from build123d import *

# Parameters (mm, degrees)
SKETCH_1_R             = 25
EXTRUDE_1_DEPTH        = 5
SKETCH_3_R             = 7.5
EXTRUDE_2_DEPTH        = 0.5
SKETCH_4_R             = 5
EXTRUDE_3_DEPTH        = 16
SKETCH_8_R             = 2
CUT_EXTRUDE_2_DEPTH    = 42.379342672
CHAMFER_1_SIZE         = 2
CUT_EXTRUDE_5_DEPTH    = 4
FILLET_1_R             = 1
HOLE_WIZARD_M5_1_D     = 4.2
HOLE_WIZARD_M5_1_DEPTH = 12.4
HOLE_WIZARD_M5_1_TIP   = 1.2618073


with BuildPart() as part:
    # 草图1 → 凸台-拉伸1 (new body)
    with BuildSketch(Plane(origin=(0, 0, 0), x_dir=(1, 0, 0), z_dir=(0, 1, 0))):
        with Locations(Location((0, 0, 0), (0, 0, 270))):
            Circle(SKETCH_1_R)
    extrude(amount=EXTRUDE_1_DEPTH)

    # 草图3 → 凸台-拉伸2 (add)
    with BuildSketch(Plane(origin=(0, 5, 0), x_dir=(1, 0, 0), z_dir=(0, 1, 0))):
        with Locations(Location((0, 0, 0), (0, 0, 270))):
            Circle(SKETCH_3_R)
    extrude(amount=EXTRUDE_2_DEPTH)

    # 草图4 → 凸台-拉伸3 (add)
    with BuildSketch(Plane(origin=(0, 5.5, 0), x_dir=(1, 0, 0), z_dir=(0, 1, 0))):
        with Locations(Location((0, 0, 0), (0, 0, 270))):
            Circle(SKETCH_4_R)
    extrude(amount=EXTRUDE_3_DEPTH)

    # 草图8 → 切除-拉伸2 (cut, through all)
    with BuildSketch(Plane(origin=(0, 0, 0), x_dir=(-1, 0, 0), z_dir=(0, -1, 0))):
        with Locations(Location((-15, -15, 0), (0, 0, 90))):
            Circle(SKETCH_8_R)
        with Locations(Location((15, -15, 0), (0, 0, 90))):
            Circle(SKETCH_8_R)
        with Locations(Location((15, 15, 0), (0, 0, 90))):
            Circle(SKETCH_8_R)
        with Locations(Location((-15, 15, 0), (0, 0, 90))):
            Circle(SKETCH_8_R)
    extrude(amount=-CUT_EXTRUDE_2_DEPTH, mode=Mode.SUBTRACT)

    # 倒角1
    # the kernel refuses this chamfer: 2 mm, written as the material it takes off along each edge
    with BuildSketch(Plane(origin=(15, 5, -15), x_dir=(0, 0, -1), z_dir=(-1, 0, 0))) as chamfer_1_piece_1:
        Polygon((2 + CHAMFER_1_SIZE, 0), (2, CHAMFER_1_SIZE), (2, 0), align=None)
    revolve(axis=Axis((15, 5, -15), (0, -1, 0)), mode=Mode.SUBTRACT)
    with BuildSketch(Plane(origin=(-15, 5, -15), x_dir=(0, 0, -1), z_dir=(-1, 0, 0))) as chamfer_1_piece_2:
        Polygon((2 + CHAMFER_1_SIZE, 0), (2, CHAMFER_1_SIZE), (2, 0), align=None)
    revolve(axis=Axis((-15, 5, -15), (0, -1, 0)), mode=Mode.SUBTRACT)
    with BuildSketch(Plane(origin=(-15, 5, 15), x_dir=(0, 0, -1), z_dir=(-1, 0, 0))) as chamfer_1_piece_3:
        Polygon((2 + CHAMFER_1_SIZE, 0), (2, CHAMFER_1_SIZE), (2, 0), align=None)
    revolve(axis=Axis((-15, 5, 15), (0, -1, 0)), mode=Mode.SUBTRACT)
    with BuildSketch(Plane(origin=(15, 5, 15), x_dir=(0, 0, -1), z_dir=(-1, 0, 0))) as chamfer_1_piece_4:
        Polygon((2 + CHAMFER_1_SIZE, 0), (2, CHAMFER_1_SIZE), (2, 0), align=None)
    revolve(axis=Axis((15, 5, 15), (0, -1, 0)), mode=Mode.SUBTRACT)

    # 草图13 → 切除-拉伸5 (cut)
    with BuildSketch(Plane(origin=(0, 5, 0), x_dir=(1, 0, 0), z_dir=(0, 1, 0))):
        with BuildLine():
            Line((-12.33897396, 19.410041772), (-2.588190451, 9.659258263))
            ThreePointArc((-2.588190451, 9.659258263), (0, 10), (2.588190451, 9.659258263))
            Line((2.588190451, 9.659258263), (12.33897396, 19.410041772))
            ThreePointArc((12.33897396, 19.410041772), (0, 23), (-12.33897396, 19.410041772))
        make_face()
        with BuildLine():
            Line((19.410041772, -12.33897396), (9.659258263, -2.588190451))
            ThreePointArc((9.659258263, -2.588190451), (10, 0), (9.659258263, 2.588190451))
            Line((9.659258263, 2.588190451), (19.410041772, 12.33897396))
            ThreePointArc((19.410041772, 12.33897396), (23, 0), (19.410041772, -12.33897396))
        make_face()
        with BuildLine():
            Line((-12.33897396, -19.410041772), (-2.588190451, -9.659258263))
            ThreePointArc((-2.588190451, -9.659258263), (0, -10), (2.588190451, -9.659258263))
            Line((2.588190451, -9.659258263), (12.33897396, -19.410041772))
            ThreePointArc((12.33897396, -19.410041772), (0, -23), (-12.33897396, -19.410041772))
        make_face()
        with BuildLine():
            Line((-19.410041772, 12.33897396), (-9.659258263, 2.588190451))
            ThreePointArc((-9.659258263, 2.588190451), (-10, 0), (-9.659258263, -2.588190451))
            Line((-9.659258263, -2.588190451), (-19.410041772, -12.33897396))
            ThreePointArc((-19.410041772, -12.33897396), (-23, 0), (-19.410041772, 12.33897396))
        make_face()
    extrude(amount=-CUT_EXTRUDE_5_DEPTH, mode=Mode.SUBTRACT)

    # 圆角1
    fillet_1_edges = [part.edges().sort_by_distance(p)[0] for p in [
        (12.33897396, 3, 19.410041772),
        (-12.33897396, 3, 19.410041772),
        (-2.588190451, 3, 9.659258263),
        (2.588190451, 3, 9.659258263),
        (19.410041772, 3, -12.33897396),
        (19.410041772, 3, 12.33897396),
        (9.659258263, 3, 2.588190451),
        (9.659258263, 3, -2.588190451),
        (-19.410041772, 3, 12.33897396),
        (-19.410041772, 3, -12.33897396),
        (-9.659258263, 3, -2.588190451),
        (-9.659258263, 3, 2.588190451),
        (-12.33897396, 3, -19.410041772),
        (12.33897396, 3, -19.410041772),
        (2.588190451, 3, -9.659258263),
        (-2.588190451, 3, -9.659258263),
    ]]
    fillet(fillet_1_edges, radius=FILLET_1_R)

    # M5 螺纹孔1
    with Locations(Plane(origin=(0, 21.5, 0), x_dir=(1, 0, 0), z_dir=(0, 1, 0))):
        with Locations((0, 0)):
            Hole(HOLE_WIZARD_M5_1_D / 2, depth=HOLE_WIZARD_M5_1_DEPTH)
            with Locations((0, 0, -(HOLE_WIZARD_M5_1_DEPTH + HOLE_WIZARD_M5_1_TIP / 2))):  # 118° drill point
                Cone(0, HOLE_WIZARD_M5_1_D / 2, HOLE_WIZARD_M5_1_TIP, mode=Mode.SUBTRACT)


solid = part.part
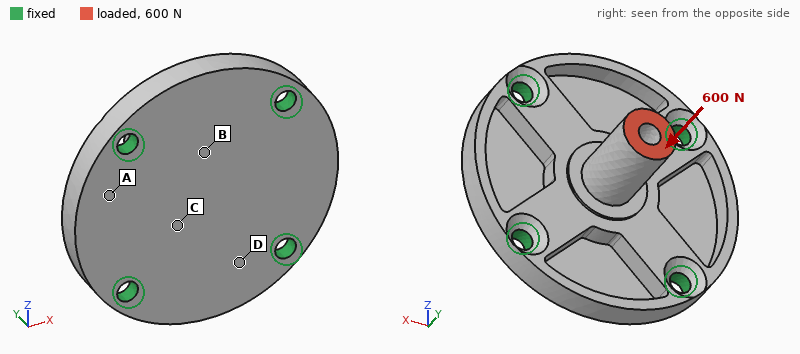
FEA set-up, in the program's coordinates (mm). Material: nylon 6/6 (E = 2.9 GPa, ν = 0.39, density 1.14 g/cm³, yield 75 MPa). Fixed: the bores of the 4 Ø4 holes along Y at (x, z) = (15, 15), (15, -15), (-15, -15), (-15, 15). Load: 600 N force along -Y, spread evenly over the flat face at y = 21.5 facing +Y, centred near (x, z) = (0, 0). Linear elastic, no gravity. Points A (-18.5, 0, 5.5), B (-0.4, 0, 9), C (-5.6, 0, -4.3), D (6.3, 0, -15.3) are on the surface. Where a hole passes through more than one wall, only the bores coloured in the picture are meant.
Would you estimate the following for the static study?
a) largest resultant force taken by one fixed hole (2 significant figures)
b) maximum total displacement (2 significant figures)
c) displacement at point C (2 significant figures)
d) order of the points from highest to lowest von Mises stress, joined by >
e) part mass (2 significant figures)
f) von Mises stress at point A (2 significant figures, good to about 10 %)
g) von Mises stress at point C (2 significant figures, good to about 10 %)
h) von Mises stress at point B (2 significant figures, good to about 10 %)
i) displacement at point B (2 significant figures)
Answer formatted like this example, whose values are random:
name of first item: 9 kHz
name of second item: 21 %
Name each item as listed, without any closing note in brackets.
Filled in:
largest resultant force taken by one fixed hole: 170 N
maximum total displacement: 0.28 mm
displacement at point C: 0.21 mm
order of the points from highest to lowest von Mises stress, joined by >: B > C > D > A
part mass: 8.4 g
von Mises stress at point A: 3.6 MPa
von Mises stress at point C: 13 MPa
von Mises stress at point B: 16 MPa
displacement at point B: 0.20 mm
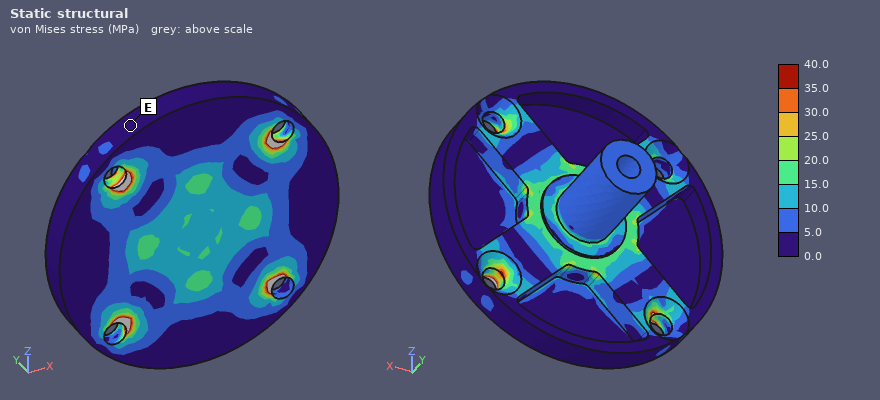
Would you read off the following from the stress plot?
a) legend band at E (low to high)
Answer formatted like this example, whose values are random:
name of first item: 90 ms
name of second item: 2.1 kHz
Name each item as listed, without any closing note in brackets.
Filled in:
legend band at E: 0.0 to 5.0 MPa
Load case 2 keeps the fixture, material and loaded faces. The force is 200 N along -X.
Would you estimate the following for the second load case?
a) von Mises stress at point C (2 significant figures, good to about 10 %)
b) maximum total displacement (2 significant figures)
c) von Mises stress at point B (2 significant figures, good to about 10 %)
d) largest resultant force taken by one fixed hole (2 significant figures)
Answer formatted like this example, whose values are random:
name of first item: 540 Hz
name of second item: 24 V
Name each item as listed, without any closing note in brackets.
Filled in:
von Mises stress at point C: 9.7 MPa
maximum total displacement: 0.58 mm
von Mises stress at point B: 6.3 MPa
largest resultant force taken by one fixed hole: 98 N
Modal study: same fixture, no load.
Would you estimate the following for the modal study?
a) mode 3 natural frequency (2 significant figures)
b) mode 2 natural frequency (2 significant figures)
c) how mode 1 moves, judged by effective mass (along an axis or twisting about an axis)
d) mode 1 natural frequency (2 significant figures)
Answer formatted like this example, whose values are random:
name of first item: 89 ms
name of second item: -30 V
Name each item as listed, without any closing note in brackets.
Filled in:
mode 3 natural frequency: 4500 Hz
mode 2 natural frequency: 4500 Hz
how mode 1 moves, judged by effective mass: along Y
mode 1 natural frequency: 4300 Hz
